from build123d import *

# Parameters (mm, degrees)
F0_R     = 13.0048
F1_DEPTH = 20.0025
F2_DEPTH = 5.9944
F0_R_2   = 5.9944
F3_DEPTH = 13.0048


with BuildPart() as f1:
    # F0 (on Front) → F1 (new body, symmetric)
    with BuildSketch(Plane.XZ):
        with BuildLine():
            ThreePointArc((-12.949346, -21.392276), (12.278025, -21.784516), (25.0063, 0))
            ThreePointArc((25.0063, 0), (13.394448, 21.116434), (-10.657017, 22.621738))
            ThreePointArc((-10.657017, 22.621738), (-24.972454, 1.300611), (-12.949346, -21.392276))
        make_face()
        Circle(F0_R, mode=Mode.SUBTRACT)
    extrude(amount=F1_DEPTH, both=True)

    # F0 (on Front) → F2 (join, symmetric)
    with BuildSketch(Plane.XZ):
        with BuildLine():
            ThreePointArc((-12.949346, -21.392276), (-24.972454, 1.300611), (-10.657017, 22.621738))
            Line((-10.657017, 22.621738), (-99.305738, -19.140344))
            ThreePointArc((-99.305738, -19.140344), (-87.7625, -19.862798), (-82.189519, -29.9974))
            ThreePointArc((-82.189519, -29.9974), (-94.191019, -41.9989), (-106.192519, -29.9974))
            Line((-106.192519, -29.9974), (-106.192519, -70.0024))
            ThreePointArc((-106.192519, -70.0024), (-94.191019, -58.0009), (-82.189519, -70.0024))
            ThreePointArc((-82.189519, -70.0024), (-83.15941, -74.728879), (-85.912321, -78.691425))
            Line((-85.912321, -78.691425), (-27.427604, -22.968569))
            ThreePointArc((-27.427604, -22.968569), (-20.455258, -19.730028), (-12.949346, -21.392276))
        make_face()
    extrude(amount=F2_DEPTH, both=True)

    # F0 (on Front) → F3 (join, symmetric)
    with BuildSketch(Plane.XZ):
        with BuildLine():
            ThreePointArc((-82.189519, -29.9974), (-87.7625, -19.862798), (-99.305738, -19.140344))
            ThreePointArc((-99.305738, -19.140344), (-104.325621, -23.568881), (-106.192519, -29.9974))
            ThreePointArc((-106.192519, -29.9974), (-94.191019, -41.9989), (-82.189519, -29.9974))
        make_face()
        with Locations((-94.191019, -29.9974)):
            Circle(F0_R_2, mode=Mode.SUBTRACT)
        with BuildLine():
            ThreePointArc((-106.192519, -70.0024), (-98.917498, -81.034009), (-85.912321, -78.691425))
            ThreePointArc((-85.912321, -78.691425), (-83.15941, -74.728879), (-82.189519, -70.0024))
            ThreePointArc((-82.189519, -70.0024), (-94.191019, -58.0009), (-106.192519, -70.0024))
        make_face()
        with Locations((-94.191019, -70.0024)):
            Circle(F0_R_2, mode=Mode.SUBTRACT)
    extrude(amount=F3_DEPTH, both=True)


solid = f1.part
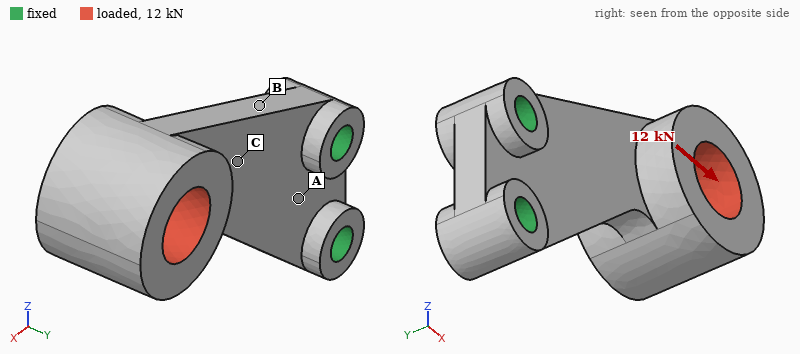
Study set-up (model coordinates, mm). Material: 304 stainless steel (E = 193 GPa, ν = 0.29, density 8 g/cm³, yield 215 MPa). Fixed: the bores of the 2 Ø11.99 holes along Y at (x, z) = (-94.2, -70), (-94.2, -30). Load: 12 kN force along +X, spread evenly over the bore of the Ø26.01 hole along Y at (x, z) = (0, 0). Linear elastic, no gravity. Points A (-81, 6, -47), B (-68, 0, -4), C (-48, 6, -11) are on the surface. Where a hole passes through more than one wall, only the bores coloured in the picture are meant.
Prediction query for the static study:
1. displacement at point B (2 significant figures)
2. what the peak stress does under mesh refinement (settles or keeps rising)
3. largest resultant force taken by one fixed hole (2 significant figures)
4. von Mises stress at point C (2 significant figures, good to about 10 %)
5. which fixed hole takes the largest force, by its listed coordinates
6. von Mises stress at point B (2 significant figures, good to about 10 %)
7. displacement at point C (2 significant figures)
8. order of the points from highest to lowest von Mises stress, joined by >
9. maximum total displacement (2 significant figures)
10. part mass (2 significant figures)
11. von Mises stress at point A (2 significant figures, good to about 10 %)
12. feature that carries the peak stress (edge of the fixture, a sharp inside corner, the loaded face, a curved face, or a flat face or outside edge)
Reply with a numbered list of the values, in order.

1. 0.025 mm
2. keeps rising
3. 19 kN
4. 46 MPa
5. (-94.2, -30)
6. 96 MPa
7. 0.031 mm
8. B > C > A
9. 0.12 mm
10. 940 g
11. 16 MPa
12. a sharp inside corner
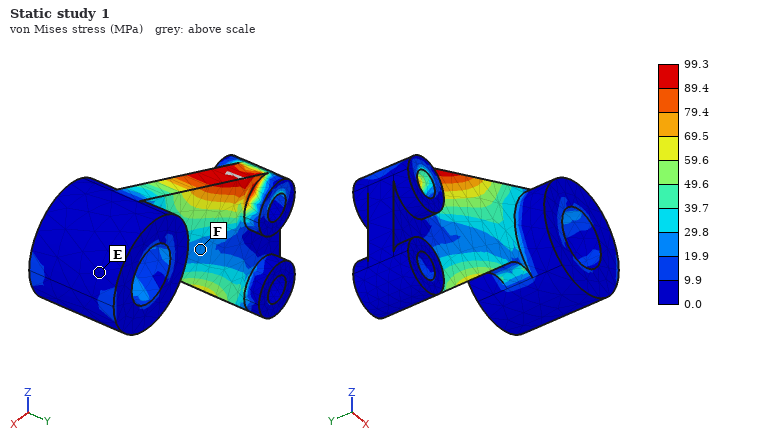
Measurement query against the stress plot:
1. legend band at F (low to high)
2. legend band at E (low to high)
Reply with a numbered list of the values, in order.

1. 19.9 to 29.8 MPa
2. 0.0 to 9.9 MPa
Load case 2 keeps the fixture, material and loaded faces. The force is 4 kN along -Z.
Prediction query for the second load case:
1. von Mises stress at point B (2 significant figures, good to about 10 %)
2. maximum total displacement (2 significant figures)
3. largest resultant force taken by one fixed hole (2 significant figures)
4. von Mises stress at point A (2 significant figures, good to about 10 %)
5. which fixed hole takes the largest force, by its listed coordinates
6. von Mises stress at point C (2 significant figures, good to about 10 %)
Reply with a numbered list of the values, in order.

1. 61 MPa
2. 0.12 mm
3. 9.1 kN
4. 22 MPa
5. (-94.2, -70)
6. 15 MPa
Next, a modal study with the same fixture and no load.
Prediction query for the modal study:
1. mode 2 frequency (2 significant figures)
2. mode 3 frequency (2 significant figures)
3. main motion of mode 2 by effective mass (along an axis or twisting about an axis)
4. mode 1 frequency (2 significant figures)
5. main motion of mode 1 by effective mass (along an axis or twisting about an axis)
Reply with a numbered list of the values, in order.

1. 1500 Hz
2. 1800 Hz
3. along Z
4. 470 Hz
5. along Y
